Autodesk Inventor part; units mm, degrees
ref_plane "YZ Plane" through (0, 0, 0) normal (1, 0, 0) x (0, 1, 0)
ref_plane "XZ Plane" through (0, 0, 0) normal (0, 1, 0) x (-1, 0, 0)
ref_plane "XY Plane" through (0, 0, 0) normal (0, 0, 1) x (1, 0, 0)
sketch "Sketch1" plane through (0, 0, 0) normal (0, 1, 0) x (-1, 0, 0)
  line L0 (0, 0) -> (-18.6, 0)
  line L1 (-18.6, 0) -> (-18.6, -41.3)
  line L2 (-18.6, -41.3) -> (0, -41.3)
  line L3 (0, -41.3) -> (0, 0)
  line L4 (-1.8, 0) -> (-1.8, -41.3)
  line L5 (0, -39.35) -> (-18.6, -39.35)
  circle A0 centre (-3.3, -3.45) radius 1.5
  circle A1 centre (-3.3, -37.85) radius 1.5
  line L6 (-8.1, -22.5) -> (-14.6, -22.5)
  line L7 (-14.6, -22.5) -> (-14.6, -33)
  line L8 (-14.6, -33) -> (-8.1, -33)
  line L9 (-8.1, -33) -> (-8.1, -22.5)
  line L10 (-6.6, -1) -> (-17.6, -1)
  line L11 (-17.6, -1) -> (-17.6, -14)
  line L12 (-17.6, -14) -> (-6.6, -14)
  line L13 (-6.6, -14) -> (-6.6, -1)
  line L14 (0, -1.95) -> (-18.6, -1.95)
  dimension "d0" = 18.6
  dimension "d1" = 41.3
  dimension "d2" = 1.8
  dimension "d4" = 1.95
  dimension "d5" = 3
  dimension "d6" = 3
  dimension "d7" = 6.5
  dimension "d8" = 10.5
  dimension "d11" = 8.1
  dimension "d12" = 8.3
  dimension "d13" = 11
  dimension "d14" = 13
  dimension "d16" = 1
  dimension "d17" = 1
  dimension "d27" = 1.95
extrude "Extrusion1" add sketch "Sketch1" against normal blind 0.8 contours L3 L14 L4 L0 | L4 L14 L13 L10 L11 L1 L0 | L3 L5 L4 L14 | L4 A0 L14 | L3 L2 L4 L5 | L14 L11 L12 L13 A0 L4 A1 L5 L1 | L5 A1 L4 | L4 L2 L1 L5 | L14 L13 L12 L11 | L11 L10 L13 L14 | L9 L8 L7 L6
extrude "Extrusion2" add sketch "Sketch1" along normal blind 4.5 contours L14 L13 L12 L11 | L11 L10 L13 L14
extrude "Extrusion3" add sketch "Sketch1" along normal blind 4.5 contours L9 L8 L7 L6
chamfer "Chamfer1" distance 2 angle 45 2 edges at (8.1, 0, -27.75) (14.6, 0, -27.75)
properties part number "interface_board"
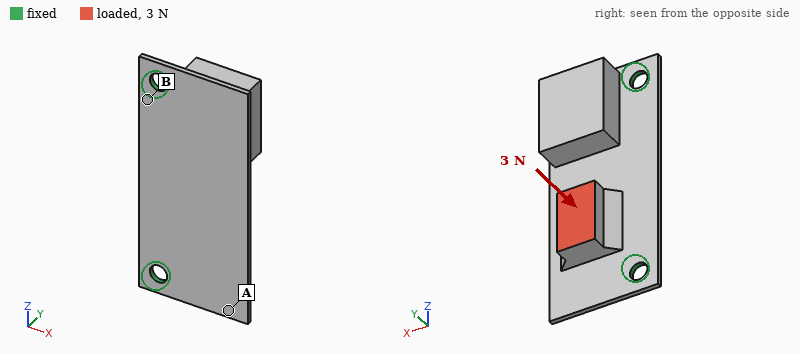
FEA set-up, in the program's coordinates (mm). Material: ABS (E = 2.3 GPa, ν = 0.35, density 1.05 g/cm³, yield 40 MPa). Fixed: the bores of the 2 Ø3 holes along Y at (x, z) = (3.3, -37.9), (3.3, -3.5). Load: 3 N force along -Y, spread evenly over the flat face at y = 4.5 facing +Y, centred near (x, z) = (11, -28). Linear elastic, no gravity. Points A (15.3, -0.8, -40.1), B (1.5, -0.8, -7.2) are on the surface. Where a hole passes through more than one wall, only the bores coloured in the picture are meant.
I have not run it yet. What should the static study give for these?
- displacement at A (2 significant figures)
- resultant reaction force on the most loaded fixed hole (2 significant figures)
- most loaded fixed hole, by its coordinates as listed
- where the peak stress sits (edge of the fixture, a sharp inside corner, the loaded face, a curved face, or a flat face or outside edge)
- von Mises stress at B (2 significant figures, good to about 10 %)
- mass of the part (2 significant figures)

0.24 mm
2.0 N
(3.3, -37.9)
a flat face or outside edge
4.0 MPa
1.7 g
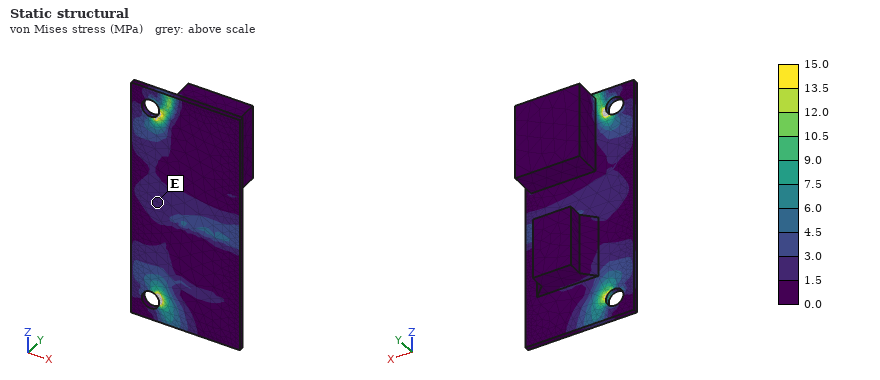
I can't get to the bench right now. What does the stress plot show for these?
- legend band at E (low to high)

1.5 to 3.0 MPa
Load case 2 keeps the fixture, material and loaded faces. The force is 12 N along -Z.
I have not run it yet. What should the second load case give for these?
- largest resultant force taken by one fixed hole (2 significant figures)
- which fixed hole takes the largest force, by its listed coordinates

7.7 N
(3.3, -37.9)
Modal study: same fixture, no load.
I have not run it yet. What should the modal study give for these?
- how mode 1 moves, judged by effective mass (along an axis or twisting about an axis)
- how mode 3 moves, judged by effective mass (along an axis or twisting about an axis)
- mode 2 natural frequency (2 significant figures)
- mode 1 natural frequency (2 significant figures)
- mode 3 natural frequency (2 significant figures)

along Y
twisting about X
1100 Hz
410 Hz
1200 Hz
